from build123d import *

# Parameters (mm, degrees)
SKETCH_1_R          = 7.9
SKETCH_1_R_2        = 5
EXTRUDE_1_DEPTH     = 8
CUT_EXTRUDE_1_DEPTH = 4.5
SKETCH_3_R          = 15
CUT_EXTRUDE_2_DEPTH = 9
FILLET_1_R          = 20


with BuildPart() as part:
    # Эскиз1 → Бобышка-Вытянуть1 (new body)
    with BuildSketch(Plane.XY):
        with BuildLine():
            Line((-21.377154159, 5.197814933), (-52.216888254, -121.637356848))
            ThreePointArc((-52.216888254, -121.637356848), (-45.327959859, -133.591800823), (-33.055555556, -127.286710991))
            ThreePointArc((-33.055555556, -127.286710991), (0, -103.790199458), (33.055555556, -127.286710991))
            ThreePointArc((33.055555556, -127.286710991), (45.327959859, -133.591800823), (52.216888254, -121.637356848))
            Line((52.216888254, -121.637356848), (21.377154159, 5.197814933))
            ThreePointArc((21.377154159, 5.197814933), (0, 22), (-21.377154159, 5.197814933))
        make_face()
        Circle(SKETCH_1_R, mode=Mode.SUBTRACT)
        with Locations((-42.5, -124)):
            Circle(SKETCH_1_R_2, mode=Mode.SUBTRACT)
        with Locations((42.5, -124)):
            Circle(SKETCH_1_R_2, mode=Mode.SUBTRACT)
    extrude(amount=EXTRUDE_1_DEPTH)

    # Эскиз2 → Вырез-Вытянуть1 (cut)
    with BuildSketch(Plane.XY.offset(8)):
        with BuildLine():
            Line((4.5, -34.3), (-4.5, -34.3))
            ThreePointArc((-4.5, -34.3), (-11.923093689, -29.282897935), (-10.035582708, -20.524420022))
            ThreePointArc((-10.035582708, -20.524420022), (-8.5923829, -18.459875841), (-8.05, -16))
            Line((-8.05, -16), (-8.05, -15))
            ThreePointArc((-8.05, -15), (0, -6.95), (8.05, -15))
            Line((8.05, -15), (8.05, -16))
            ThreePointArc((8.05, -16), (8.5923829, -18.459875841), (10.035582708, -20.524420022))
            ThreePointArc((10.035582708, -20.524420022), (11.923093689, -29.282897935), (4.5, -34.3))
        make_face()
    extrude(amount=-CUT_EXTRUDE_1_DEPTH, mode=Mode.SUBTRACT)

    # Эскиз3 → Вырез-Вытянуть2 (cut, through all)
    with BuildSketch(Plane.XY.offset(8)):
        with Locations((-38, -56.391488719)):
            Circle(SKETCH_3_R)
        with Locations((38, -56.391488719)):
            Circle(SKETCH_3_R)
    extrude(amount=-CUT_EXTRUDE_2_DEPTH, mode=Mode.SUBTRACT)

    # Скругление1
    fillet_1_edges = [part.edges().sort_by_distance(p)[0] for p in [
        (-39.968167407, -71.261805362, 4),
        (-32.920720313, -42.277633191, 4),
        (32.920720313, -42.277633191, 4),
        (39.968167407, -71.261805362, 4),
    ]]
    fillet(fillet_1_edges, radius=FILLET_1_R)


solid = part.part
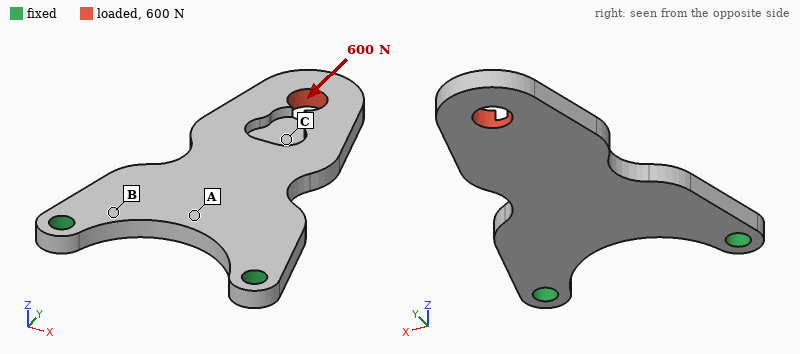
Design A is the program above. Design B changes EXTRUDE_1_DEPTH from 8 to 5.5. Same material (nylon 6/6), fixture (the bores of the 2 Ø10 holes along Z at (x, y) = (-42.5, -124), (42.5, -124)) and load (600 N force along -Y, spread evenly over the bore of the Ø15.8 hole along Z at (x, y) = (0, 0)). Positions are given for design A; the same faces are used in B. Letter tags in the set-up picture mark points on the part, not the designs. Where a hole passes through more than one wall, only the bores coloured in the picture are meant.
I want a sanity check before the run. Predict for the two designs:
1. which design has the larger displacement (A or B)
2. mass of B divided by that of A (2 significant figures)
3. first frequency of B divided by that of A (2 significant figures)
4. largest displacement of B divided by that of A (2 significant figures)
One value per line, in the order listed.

B
0.70
0.69
1.4
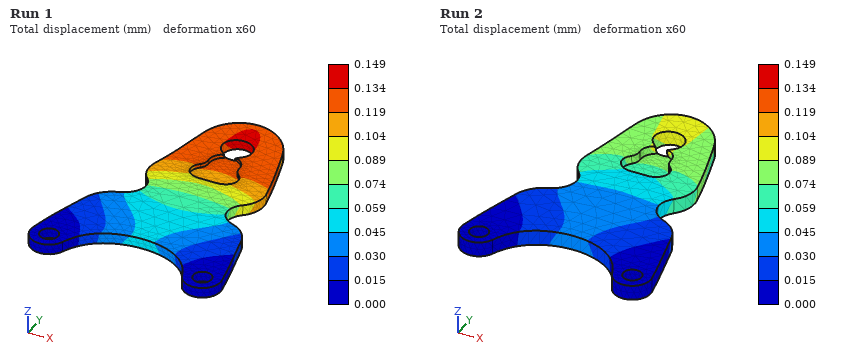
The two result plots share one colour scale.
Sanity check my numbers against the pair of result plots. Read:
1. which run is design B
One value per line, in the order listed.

Run 1
